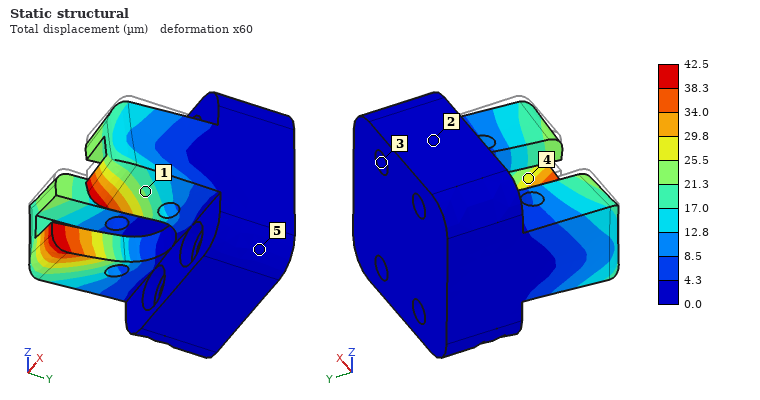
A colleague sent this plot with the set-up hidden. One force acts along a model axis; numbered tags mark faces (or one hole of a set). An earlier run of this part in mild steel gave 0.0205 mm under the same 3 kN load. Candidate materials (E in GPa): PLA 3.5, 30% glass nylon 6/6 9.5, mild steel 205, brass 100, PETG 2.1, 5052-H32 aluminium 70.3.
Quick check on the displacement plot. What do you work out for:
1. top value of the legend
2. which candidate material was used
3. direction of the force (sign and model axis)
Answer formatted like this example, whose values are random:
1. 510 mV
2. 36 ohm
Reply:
1. 42.5 µm
2. brass
3. -Z
